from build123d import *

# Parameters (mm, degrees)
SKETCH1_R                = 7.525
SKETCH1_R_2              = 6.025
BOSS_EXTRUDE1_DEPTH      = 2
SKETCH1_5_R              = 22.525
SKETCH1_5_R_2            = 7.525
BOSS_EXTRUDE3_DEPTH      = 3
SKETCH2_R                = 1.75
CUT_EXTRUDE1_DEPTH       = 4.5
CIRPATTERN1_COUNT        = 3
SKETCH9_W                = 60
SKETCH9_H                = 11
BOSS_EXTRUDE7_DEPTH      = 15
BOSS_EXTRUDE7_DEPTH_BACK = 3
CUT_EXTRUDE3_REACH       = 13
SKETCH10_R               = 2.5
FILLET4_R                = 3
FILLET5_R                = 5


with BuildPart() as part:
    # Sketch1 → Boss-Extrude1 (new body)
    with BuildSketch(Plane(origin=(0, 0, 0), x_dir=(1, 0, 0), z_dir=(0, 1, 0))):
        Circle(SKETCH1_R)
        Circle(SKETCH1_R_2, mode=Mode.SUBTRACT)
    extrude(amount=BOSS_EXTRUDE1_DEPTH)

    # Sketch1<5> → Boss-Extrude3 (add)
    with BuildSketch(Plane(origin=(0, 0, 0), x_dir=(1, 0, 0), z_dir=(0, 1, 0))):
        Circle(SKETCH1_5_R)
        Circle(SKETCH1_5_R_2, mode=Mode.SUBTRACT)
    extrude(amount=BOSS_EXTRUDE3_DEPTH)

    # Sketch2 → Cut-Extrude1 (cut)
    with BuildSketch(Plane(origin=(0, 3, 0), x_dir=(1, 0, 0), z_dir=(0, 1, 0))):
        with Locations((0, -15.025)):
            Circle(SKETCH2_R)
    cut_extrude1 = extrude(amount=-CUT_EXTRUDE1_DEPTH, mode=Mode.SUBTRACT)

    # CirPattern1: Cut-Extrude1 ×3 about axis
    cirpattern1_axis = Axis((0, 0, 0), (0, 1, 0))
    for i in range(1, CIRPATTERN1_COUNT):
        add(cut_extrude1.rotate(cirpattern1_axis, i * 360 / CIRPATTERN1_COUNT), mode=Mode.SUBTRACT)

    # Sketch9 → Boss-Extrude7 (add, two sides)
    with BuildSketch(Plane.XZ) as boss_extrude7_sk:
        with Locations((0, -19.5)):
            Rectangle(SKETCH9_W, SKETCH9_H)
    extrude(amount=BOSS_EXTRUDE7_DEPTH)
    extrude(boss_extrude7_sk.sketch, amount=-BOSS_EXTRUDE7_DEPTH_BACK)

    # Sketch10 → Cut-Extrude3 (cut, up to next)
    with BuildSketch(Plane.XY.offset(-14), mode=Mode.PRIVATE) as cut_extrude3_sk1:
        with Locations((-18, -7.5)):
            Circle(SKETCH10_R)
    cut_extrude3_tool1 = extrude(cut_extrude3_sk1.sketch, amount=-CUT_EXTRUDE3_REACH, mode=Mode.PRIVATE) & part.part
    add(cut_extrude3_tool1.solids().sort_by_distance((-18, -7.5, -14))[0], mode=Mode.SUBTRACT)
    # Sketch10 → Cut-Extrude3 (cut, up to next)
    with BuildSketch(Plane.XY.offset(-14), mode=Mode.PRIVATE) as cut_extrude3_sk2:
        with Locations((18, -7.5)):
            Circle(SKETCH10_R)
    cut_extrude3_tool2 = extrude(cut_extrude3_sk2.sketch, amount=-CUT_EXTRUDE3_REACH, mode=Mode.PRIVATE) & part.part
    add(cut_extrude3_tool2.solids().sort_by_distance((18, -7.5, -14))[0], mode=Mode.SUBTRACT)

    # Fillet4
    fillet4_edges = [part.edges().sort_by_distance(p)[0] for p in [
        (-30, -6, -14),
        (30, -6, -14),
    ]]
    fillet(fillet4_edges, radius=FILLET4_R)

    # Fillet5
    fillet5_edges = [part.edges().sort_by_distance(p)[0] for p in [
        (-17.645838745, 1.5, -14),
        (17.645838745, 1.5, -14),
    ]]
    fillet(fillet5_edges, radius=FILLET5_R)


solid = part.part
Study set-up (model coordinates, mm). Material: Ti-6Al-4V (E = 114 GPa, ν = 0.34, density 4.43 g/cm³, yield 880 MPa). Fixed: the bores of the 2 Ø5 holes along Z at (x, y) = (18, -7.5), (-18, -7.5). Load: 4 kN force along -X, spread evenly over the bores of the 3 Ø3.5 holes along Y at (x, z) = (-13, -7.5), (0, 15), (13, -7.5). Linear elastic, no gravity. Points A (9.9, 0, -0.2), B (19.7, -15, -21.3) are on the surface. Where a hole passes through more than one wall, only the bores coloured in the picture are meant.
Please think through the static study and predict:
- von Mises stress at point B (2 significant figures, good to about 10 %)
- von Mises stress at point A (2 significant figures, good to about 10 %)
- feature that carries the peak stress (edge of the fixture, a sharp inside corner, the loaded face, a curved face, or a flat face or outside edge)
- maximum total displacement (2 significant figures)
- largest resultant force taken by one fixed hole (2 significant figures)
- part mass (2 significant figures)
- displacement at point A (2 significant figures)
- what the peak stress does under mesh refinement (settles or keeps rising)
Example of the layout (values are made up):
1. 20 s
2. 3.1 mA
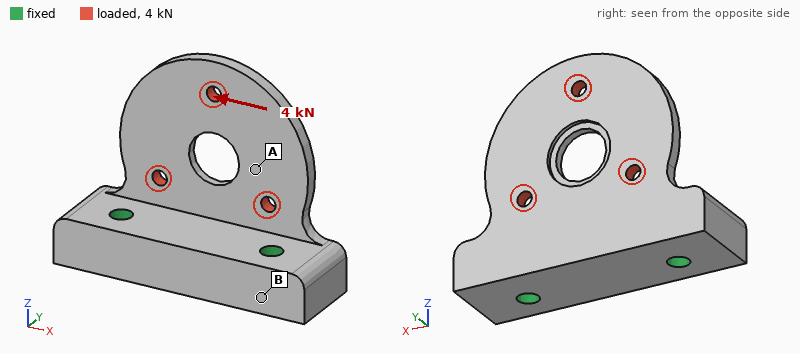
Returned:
1. 14 MPa
2. 42 MPa
3. a sharp inside corner
4. 39 µm
5. 2.9 kN
6. 67 g
7. 21 µm
8. keeps rising
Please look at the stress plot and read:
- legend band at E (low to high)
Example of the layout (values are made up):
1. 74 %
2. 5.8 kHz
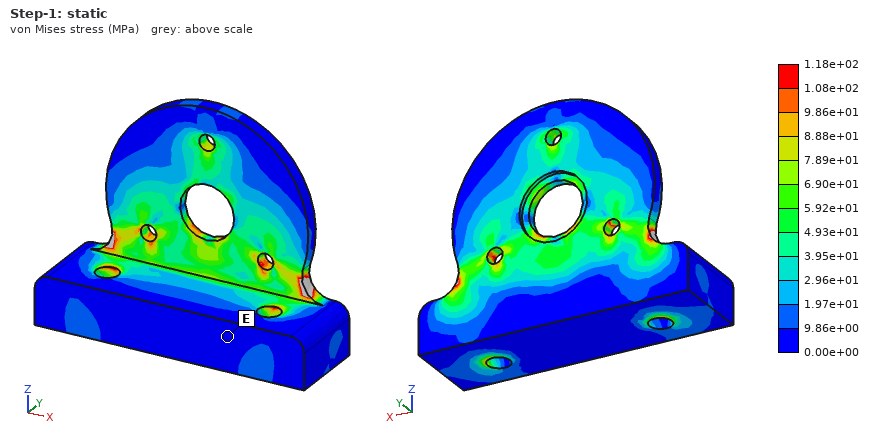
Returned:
1. 0.00e+00 to 9.86e+00 MPa
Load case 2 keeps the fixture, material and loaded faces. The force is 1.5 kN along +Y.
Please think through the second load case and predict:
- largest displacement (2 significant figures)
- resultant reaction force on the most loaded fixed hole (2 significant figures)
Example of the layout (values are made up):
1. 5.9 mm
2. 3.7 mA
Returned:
1. 0.88 mm
2. 780 N
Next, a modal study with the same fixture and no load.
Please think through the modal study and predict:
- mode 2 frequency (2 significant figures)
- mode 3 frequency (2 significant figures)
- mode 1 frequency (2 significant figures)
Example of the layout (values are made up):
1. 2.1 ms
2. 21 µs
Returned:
1. 4700 Hz
2. 9800 Hz
3. 1900 Hz
